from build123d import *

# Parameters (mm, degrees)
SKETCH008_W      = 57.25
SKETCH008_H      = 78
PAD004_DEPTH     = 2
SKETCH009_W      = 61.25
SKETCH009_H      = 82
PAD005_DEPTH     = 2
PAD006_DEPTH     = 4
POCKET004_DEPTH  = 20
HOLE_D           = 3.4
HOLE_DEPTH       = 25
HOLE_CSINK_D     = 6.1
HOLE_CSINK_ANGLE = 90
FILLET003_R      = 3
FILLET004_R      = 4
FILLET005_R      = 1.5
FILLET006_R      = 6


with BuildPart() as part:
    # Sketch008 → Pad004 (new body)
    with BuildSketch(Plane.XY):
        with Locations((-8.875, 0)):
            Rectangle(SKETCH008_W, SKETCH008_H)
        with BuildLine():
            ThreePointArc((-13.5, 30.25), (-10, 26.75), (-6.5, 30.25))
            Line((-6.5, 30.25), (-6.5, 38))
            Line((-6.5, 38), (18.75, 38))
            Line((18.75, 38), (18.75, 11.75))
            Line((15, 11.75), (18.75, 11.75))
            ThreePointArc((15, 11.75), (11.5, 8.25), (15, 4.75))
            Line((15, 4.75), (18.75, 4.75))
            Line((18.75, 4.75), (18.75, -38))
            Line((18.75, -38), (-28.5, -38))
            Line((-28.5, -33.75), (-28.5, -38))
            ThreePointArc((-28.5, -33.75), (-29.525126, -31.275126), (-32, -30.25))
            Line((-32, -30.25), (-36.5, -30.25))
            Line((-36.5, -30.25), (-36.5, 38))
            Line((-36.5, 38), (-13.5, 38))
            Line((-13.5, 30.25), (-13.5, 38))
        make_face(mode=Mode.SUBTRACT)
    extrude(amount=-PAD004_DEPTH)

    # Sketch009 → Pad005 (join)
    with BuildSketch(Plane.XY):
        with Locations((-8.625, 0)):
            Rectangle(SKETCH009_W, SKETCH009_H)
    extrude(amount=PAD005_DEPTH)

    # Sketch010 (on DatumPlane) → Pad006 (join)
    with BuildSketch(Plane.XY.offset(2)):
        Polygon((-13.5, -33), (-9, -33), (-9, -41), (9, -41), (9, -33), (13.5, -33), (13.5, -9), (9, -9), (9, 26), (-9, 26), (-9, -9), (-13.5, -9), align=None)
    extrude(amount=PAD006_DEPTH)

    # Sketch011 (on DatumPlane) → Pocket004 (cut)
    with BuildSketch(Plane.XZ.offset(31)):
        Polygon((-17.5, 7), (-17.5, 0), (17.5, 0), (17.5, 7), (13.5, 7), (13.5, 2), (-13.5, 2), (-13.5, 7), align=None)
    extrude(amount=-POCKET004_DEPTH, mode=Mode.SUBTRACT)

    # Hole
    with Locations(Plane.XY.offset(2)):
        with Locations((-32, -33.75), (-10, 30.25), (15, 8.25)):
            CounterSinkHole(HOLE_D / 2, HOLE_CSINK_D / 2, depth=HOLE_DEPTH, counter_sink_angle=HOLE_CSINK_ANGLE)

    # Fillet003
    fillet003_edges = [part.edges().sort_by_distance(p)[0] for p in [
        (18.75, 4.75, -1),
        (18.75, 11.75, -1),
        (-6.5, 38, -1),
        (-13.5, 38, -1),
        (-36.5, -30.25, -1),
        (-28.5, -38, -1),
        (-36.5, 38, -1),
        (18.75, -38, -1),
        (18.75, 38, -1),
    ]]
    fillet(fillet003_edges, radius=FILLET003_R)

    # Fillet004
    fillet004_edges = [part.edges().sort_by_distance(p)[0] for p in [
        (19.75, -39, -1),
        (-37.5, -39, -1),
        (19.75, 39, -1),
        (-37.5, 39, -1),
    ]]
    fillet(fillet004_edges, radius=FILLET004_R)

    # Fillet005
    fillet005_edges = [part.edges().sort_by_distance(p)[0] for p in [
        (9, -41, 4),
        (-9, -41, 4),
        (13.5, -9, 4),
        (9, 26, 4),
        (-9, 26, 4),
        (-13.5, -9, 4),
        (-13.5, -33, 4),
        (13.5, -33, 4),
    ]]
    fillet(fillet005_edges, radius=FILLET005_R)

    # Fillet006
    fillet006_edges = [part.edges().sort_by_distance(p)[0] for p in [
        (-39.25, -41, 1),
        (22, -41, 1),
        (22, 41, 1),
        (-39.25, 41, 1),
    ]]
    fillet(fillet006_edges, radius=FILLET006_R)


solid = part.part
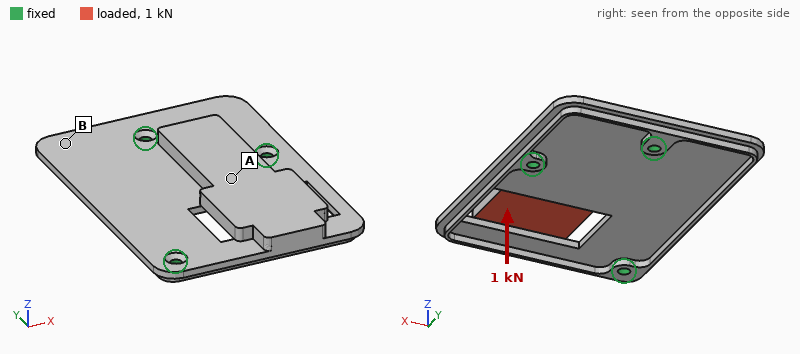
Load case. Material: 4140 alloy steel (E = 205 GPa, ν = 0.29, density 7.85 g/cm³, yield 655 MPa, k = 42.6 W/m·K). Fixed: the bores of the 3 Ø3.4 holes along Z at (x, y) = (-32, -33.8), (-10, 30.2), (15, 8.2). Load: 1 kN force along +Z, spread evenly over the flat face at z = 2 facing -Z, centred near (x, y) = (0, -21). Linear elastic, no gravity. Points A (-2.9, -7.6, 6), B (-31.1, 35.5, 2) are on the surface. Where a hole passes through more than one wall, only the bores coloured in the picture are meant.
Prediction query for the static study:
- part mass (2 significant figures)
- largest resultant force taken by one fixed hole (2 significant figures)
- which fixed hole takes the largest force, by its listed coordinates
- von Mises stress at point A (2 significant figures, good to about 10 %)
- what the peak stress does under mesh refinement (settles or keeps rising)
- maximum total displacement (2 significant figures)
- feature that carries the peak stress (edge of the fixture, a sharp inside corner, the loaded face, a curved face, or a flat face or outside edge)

120 g
1.6 kN
(15, 8.2)
57 MPa
keeps rising
0.18 mm
a sharp inside corner
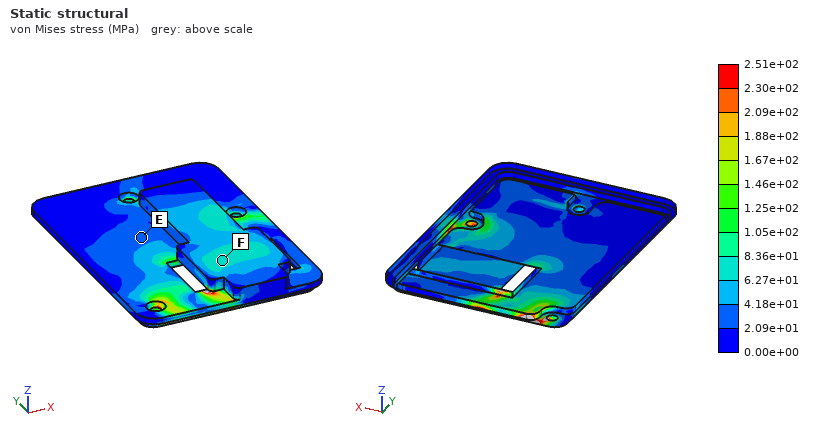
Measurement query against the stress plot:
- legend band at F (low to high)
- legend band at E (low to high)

6.27e+01 to 8.36e+01 MPa
2.09e+01 to 4.18e+01 MPa
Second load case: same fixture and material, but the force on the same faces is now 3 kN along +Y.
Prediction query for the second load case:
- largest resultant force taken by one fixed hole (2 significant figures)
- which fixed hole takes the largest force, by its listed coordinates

1.3 kN
(15, 8.2)
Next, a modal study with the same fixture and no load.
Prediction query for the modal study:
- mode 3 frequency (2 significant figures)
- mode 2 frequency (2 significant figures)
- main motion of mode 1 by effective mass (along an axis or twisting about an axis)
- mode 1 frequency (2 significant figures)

3900 Hz
2300 Hz
along Z
2100 Hz
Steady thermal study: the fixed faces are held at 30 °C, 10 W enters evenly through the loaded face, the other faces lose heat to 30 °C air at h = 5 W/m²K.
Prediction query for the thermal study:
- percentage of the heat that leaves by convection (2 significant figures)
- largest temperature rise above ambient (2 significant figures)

10 %
48 K
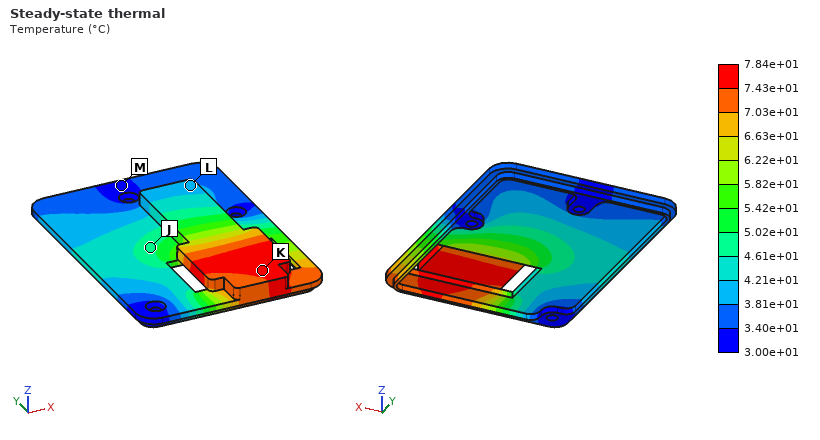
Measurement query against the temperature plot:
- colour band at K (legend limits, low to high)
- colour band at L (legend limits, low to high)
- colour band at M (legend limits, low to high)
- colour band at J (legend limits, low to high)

7.43e+01 to 7.84e+01 °C
3.81e+01 to 4.21e+01 °C
3.00e+01 to 3.40e+01 °C
4.61e+01 to 5.02e+01 °C
